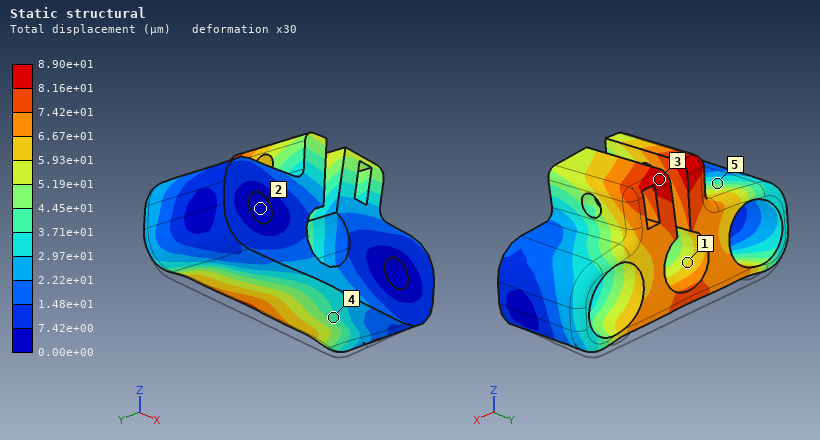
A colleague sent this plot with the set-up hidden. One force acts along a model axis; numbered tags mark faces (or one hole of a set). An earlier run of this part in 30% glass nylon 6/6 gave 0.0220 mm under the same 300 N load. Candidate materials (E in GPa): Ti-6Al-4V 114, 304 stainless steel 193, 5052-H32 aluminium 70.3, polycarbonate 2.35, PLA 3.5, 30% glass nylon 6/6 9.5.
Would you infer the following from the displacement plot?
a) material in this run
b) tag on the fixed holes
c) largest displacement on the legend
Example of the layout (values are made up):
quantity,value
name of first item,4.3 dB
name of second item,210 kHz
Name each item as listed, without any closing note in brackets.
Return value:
quantity,value
material in this run,polycarbonate
tag on the fixed holes,2
largest displacement on the legend,8.90e+01 µm
